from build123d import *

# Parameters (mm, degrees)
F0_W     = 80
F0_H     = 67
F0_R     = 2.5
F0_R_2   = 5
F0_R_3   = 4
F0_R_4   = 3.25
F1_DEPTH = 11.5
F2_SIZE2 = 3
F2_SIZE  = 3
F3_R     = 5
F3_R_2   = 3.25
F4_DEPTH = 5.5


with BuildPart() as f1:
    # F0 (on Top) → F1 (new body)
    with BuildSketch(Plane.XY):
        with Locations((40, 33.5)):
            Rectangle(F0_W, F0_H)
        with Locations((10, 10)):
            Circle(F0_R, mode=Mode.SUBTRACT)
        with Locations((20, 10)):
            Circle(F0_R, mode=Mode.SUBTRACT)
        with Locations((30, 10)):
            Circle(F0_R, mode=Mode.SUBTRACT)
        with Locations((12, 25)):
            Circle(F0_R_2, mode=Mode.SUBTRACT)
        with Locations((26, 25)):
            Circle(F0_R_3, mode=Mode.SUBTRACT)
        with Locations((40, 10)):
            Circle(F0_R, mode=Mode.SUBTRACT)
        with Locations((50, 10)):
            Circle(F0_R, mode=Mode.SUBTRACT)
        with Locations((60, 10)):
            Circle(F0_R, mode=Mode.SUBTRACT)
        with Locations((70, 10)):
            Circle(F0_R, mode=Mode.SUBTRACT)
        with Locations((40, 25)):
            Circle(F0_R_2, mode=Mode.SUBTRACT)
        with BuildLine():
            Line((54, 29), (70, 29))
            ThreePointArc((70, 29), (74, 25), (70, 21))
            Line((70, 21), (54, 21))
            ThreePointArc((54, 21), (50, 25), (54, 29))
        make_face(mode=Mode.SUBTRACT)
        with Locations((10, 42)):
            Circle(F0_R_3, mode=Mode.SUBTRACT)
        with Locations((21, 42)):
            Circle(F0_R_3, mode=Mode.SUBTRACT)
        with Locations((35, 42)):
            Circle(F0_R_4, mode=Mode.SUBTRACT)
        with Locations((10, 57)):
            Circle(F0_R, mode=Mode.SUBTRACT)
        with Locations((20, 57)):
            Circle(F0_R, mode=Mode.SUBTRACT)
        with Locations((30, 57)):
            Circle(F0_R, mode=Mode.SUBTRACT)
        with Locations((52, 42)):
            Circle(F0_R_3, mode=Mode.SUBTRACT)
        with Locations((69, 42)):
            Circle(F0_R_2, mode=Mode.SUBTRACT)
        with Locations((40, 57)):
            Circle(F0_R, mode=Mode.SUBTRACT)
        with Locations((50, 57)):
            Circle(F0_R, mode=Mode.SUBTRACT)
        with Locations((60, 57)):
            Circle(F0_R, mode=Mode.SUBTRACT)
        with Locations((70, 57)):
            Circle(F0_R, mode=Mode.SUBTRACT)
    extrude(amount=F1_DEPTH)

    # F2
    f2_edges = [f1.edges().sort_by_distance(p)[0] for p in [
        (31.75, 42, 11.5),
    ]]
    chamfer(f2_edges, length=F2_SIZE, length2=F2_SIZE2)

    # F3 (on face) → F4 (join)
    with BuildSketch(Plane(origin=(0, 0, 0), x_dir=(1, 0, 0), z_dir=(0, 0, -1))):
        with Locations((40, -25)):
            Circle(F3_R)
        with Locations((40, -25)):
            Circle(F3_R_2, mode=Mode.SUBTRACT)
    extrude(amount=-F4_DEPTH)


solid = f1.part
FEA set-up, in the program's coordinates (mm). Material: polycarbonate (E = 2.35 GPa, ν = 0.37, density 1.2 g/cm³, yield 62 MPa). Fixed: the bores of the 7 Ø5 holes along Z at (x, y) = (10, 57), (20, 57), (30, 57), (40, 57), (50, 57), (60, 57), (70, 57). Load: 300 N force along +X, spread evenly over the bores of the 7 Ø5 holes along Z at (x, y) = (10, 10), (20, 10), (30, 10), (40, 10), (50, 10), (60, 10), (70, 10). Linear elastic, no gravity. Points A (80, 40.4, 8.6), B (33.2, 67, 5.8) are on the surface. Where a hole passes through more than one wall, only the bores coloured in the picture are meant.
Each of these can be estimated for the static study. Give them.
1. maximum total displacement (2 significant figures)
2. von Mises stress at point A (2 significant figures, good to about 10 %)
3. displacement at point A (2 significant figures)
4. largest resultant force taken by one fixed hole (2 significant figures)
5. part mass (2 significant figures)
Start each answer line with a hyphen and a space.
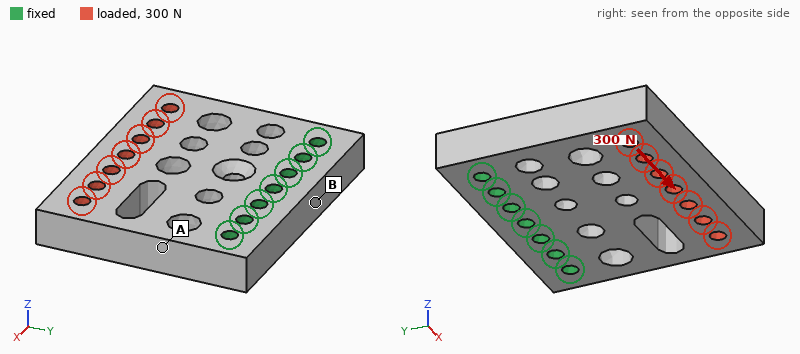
- 69 µm
- 1.00 MPa
- 21 µm
- 190 N
- 61 g
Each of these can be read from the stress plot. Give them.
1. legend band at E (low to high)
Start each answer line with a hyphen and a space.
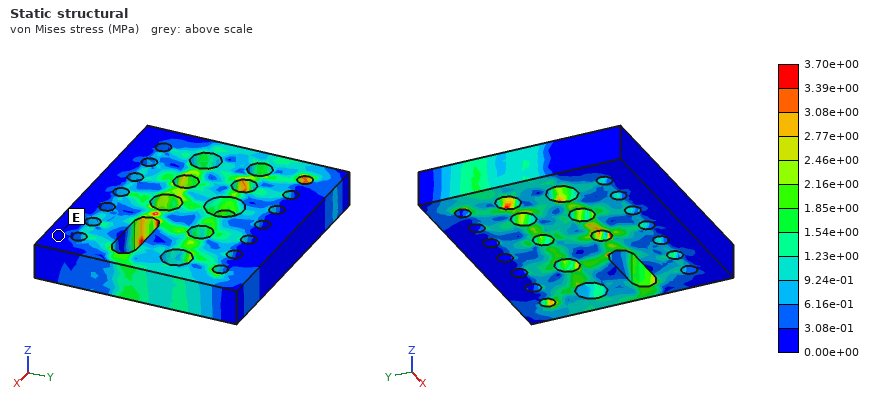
- 0.00e+00 to 3.08e-01 MPa
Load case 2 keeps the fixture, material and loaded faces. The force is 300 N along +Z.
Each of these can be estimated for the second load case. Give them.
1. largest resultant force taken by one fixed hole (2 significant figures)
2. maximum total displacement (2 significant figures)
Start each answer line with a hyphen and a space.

- 59 N
- 0.86 mm
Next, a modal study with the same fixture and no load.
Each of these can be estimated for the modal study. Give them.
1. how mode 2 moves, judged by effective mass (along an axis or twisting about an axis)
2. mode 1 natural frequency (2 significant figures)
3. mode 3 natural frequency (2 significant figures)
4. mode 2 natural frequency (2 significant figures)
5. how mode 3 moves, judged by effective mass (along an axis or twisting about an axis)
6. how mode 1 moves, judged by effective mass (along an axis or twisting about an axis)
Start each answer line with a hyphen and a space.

- twisting about Y
- 720 Hz
- 2200 Hz
- 1200 Hz
- along X
- along Z
